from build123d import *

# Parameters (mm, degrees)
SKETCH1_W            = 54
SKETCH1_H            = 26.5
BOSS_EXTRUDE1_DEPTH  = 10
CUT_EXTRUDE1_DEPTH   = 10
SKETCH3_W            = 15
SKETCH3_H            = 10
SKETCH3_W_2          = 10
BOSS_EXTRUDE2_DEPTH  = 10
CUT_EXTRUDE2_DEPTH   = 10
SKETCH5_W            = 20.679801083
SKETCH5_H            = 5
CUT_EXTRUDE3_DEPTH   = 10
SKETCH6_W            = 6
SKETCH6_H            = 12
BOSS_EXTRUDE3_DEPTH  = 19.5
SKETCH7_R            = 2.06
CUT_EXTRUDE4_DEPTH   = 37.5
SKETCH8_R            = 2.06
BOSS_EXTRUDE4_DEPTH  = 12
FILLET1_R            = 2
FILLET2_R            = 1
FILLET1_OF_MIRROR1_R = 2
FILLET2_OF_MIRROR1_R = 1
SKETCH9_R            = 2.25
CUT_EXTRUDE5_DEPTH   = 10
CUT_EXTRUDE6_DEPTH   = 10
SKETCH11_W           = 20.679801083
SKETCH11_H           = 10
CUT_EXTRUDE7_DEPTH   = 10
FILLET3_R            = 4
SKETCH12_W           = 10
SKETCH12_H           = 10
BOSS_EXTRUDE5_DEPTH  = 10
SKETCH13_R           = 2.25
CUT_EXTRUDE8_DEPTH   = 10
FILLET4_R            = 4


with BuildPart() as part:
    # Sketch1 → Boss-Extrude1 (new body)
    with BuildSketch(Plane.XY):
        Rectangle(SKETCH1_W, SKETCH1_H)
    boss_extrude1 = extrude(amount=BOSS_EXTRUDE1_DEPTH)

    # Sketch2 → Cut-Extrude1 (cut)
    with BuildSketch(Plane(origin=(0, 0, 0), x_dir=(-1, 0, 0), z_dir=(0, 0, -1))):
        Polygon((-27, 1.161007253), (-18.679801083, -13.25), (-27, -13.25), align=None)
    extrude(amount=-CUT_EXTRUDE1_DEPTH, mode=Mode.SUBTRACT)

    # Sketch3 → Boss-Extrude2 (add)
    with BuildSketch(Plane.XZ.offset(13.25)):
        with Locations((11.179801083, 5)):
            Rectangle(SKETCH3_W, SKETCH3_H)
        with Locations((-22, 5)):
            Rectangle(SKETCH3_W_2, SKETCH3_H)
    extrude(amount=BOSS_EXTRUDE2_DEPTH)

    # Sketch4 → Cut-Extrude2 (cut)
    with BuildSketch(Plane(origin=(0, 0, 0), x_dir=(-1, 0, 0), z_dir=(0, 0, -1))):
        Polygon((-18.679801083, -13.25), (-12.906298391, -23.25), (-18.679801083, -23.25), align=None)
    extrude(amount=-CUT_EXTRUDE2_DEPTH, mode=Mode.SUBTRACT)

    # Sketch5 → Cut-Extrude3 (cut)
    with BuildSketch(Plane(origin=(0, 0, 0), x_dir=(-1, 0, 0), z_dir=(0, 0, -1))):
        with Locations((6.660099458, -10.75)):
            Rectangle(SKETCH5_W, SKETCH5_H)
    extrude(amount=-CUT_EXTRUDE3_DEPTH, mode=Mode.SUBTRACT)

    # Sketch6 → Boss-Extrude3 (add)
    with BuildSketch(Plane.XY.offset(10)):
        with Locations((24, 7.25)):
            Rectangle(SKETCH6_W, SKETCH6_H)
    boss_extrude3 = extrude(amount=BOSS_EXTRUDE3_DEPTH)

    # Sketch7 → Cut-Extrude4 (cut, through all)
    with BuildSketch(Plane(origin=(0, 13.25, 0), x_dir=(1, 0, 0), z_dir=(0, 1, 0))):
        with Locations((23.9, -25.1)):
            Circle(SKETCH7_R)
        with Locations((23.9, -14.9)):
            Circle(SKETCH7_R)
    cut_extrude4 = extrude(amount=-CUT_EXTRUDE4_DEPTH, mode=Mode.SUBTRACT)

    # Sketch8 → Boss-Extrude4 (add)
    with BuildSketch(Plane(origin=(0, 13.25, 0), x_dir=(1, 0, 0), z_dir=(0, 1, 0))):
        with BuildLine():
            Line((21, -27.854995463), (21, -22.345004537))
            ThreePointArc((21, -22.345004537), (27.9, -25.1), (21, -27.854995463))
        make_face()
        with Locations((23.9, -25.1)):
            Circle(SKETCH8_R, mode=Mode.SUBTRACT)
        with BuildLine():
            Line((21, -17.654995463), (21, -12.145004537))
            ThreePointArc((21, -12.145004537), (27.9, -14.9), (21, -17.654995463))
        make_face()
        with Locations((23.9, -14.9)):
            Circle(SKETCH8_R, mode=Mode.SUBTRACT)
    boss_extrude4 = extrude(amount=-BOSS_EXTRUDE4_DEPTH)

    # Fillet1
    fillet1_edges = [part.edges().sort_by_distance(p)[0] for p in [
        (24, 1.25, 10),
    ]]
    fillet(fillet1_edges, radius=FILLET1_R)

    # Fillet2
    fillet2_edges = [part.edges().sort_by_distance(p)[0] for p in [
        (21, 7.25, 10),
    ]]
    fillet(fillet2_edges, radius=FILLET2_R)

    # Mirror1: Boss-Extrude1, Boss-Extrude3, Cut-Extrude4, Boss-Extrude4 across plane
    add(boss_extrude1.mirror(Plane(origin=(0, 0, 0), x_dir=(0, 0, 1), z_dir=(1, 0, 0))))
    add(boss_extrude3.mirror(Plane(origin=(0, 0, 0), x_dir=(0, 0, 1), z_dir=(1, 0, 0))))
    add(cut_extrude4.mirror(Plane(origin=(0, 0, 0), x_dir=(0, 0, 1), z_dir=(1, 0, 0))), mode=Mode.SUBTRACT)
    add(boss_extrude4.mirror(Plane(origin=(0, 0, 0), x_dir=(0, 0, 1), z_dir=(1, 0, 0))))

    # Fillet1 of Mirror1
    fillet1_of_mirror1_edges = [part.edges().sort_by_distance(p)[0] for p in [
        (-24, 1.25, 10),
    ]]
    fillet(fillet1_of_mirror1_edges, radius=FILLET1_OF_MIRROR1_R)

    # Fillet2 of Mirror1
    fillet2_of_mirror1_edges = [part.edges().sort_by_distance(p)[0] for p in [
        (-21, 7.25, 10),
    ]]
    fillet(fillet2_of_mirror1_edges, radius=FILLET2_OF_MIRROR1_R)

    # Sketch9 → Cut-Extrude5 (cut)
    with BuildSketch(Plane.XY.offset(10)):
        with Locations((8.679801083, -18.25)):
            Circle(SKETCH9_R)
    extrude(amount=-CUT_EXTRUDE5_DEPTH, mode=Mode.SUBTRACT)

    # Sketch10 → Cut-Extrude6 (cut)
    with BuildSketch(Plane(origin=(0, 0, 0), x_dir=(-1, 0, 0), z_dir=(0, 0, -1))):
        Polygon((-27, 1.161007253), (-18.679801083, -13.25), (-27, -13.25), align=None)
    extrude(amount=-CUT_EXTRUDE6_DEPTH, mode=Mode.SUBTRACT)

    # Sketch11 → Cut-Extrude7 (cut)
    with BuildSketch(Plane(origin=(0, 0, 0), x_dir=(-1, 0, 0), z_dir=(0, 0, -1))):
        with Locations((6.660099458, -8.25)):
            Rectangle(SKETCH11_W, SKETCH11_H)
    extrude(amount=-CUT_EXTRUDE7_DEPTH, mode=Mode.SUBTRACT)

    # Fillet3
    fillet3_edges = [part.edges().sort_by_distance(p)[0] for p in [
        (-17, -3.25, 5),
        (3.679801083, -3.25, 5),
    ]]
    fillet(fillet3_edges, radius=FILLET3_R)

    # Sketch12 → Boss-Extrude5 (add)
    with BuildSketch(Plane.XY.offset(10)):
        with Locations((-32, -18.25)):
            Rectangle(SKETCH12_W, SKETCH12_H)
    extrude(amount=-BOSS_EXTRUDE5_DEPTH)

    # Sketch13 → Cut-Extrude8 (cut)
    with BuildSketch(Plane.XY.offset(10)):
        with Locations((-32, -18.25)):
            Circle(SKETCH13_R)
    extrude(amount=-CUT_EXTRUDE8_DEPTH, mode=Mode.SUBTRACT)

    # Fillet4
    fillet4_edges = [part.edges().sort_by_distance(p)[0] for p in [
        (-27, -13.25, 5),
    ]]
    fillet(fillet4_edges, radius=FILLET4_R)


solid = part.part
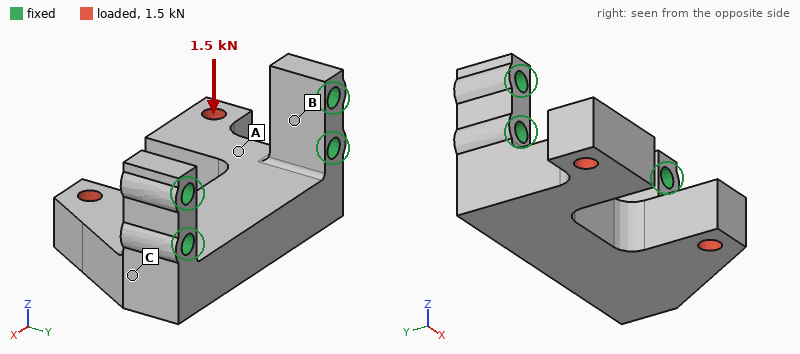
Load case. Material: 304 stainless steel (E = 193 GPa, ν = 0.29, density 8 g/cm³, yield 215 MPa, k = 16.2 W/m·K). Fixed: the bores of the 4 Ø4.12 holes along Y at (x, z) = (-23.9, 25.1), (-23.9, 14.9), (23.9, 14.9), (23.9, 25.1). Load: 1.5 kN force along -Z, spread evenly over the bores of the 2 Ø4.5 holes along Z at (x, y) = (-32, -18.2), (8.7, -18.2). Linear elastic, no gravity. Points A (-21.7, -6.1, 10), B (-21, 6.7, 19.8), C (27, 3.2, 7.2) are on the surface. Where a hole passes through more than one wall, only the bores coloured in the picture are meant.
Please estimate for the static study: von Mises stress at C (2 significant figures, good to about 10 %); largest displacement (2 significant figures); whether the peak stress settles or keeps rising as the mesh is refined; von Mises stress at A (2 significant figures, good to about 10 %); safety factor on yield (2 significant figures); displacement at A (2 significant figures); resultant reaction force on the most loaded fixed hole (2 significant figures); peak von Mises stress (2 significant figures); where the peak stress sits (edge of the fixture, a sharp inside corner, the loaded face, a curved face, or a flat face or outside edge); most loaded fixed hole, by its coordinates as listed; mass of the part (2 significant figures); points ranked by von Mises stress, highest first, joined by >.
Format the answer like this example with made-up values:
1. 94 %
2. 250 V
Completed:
1. 39 MPa
2. 62 µm
3. settles
4. 75 MPa
5. 0.58
6. 15 µm
7. 1.1 kN
8. 370 MPa
9. a curved face
10. (-23.9, 14.9)
11. 140 g
12. A > C > B
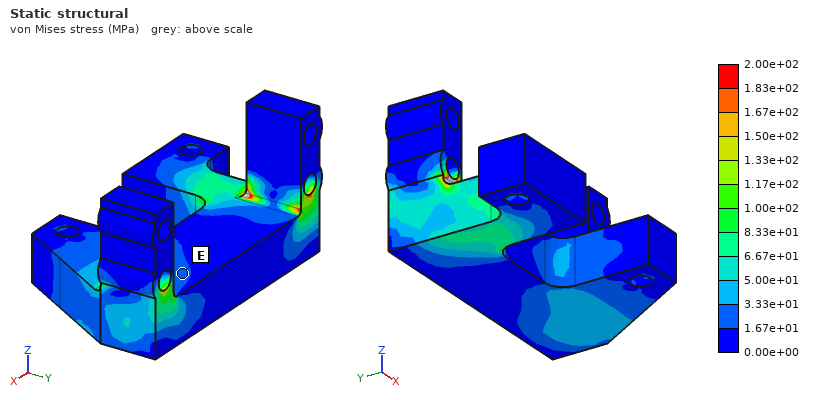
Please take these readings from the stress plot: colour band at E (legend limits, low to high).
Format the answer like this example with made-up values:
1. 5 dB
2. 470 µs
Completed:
1. 1.67e+01 to 3.33e+01 MPa
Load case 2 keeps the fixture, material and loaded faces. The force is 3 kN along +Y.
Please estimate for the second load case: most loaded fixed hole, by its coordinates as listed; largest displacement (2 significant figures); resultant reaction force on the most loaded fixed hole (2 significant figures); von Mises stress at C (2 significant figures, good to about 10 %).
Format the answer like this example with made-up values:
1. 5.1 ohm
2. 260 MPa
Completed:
1. (-23.9, 14.9)
2. 46 µm
3. 2.2 kN
4. 14 MPa
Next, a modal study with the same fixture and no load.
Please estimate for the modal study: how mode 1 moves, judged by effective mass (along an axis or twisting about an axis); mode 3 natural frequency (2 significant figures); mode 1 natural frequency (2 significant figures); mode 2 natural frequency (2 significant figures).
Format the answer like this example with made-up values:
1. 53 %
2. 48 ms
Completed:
1. along Z
2. 7700 Hz
3. 5300 Hz
4. 6800 Hz
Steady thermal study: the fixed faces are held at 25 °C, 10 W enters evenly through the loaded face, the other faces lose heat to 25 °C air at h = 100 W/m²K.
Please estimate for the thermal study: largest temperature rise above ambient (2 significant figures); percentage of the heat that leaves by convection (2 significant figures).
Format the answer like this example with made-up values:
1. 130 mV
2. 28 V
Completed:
1. 45 K
2. 77 %
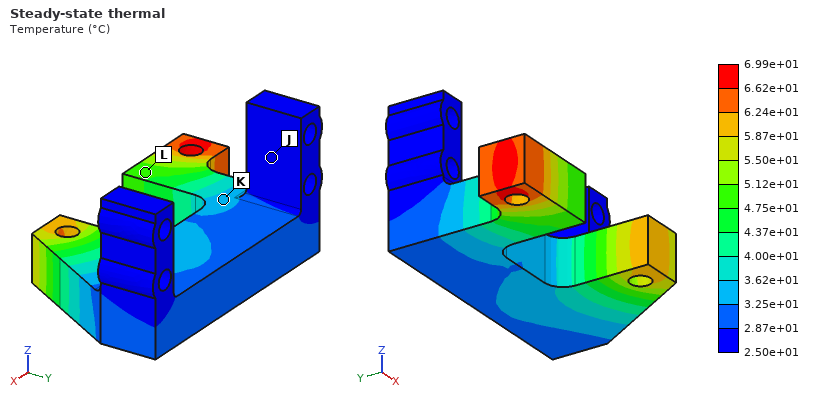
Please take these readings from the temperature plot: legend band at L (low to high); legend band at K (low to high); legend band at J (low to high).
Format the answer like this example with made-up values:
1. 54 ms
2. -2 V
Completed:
1. 4.75e+01 to 5.12e+01 °C
2. 3.25e+01 to 3.62e+01 °C
3. 2.50e+01 to 2.87e+01 °C
